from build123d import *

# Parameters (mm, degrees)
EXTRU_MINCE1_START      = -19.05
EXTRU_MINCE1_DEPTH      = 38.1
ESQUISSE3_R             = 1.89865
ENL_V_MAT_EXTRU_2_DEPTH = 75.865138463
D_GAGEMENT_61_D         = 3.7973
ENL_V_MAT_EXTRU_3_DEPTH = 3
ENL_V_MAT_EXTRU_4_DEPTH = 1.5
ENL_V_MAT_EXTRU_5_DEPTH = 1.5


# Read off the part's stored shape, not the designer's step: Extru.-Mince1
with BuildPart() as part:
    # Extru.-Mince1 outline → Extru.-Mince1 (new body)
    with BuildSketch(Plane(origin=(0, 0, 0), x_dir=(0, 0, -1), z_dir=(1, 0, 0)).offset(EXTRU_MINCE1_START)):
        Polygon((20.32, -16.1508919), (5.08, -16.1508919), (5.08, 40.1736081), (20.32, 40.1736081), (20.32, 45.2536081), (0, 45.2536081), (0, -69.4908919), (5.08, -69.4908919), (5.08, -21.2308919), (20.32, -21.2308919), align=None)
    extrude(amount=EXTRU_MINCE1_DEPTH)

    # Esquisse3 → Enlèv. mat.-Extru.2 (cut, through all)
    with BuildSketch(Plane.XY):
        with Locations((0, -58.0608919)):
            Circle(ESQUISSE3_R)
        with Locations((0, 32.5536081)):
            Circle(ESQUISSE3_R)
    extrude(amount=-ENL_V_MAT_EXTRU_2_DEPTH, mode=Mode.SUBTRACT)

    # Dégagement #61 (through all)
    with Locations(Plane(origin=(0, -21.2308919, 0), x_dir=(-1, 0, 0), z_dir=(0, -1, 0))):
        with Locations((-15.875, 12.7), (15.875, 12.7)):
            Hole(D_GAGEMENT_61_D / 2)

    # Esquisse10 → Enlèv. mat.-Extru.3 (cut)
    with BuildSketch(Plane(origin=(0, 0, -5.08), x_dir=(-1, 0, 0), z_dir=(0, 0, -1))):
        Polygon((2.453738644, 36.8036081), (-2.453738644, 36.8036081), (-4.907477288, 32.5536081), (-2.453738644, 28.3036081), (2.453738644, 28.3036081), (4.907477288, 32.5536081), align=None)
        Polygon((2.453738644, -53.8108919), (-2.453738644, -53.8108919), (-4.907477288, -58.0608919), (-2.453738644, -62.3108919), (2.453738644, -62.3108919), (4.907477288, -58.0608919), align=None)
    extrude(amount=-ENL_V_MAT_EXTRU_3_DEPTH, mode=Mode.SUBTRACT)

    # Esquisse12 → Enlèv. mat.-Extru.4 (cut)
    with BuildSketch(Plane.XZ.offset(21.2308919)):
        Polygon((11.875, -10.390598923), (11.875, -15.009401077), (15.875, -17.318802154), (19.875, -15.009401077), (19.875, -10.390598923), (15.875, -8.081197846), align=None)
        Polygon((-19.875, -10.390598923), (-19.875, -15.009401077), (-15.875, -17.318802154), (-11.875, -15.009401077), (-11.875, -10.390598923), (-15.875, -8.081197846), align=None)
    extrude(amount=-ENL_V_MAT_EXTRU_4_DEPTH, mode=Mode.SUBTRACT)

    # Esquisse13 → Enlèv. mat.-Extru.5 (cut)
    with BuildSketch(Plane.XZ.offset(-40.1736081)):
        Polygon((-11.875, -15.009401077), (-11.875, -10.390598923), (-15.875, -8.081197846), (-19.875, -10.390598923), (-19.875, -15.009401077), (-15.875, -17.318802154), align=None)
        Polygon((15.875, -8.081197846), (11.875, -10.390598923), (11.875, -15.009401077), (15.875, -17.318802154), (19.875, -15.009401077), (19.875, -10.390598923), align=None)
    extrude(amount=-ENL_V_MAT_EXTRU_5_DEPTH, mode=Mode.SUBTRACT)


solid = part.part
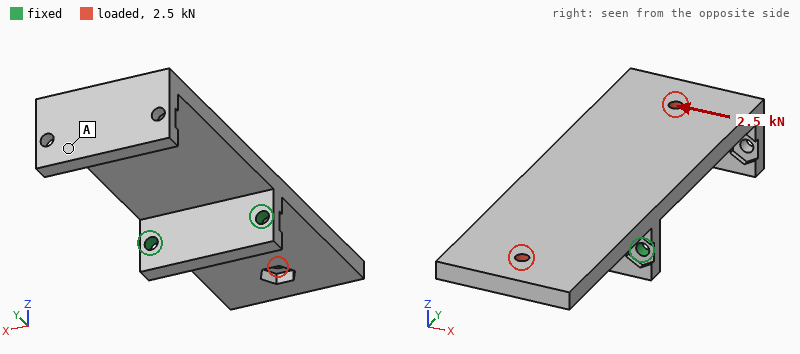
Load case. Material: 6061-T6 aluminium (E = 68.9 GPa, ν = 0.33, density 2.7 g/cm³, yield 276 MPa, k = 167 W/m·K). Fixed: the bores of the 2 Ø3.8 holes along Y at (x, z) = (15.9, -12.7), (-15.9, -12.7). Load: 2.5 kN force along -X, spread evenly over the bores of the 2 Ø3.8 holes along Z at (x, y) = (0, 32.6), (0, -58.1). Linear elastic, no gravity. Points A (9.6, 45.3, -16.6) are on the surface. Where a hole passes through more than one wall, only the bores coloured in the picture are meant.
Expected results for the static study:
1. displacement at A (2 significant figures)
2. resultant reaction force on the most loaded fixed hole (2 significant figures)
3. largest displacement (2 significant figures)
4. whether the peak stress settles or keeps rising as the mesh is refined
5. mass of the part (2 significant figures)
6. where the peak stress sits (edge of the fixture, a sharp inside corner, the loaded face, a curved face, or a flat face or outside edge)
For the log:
0.11 mm
1.6 kN
0.13 mm
keeps rising
73 g
edge of the fixture
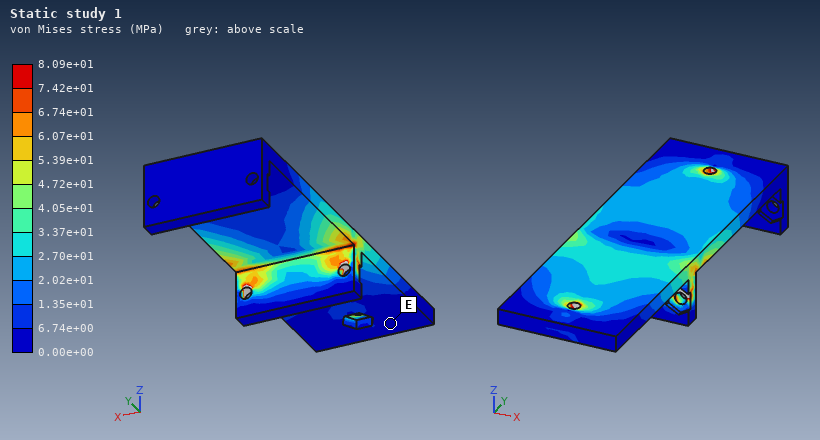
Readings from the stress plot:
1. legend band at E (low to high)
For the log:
0.00e+00 to 6.74e+00 MPa
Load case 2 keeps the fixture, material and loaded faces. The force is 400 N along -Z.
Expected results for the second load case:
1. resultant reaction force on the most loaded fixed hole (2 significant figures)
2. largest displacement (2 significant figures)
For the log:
240 N
0.50 mm
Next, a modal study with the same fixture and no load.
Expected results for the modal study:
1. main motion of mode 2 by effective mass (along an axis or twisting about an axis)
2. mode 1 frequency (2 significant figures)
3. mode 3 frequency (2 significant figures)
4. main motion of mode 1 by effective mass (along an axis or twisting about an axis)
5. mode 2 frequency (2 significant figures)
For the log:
along Z
540 Hz
1800 Hz
along Z
1300 Hz
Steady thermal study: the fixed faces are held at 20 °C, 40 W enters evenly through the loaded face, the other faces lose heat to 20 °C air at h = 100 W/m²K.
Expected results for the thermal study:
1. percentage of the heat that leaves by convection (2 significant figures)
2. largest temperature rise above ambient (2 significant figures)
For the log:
53 %
36 K
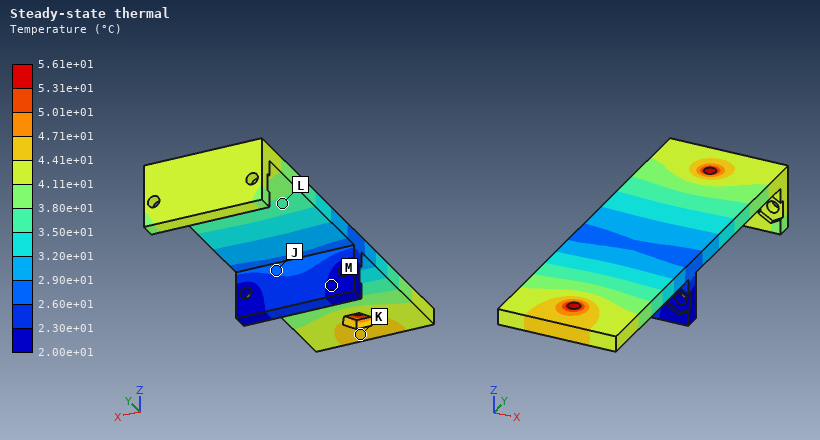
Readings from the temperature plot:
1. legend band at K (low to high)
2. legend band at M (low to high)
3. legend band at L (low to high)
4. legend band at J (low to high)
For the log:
4.41e+01 to 4.71e+01 °C
2.00e+01 to 2.30e+01 °C
3.50e+01 to 3.80e+01 °C
2.60e+01 to 2.90e+01 °C
